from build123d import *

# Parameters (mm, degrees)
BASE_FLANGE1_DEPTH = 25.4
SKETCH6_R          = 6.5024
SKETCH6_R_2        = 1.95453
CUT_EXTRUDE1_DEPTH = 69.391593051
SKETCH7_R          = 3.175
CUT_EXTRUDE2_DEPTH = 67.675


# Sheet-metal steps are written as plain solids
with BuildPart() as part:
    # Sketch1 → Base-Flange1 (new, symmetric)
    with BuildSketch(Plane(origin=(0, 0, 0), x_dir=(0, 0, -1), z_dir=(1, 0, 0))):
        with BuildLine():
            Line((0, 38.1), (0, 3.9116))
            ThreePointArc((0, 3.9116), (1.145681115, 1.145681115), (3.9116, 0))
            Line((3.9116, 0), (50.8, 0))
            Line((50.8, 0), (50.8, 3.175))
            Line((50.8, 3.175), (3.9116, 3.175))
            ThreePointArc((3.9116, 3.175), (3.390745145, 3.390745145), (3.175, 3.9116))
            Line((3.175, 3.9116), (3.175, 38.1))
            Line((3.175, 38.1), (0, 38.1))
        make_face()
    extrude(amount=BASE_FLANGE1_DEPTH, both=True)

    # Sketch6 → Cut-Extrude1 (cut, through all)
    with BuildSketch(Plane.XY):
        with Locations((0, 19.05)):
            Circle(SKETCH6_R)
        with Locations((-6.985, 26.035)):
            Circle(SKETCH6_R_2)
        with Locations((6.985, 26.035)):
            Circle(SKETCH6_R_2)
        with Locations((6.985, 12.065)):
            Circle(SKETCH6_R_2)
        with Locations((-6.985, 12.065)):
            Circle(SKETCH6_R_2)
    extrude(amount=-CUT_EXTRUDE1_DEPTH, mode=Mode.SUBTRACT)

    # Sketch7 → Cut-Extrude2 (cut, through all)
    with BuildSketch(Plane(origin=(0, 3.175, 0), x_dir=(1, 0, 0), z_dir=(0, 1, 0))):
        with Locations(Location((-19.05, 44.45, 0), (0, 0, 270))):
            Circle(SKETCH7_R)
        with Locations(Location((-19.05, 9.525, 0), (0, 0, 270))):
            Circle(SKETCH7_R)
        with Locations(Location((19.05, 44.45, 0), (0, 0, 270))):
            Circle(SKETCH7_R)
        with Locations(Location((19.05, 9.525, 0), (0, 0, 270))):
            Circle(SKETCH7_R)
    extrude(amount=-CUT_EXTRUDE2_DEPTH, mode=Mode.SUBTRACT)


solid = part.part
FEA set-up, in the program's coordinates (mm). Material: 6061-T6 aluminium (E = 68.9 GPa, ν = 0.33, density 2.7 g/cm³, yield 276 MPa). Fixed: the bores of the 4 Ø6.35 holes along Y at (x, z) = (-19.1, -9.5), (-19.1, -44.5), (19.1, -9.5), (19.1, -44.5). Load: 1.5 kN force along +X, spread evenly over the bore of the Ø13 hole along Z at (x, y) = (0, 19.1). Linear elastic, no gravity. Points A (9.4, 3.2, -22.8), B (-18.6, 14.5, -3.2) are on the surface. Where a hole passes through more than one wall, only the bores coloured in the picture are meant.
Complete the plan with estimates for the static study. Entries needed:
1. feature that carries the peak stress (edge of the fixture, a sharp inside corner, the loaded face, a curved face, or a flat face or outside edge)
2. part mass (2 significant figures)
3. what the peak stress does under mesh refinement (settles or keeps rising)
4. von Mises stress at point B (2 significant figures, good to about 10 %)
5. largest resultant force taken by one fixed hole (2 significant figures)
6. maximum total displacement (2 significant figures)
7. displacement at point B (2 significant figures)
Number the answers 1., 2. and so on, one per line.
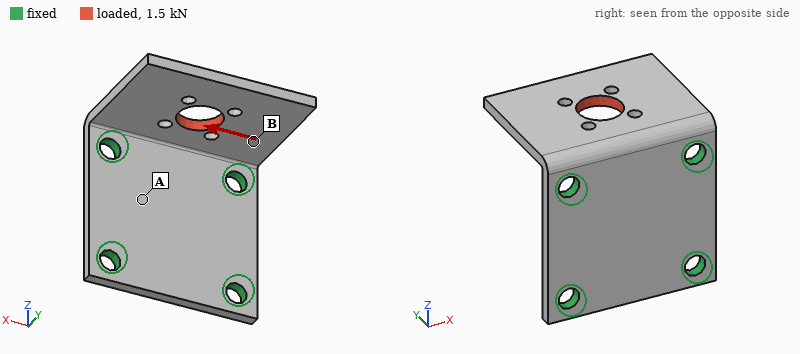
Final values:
1. edge of the fixture
2. 34 g
3. keeps rising
4. 25 MPa
5. 1.0 kN
6. 74 µm
7. 34 µm
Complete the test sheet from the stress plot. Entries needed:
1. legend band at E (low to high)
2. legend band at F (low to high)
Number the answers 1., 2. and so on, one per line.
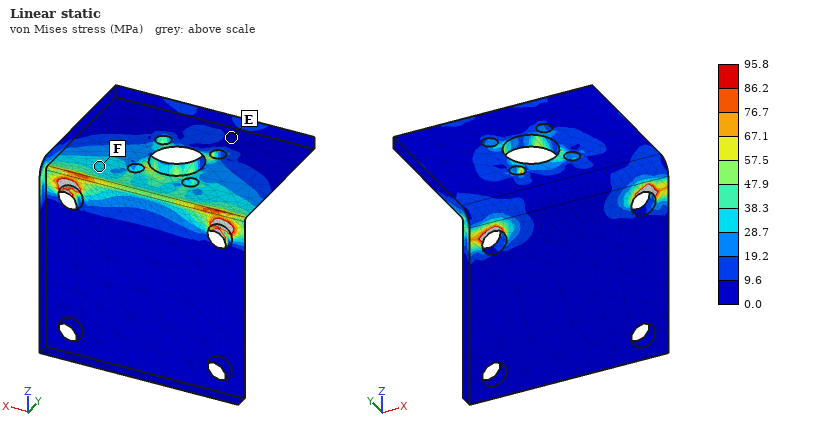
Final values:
1. 0.0 to 9.6 MPa
2. 28.7 to 38.3 MPa
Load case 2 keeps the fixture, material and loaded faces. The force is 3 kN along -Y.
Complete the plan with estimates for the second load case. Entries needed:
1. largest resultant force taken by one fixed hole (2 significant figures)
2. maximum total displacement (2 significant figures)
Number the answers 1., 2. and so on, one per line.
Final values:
1. 1.6 kN
2. 0.28 mm
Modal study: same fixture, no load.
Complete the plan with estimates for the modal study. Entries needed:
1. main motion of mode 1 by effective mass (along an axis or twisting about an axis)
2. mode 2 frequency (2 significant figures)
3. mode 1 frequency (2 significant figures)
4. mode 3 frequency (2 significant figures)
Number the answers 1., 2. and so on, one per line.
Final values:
1. along Z
2. 3100 Hz
3. 1500 Hz
4. 8000 Hz
